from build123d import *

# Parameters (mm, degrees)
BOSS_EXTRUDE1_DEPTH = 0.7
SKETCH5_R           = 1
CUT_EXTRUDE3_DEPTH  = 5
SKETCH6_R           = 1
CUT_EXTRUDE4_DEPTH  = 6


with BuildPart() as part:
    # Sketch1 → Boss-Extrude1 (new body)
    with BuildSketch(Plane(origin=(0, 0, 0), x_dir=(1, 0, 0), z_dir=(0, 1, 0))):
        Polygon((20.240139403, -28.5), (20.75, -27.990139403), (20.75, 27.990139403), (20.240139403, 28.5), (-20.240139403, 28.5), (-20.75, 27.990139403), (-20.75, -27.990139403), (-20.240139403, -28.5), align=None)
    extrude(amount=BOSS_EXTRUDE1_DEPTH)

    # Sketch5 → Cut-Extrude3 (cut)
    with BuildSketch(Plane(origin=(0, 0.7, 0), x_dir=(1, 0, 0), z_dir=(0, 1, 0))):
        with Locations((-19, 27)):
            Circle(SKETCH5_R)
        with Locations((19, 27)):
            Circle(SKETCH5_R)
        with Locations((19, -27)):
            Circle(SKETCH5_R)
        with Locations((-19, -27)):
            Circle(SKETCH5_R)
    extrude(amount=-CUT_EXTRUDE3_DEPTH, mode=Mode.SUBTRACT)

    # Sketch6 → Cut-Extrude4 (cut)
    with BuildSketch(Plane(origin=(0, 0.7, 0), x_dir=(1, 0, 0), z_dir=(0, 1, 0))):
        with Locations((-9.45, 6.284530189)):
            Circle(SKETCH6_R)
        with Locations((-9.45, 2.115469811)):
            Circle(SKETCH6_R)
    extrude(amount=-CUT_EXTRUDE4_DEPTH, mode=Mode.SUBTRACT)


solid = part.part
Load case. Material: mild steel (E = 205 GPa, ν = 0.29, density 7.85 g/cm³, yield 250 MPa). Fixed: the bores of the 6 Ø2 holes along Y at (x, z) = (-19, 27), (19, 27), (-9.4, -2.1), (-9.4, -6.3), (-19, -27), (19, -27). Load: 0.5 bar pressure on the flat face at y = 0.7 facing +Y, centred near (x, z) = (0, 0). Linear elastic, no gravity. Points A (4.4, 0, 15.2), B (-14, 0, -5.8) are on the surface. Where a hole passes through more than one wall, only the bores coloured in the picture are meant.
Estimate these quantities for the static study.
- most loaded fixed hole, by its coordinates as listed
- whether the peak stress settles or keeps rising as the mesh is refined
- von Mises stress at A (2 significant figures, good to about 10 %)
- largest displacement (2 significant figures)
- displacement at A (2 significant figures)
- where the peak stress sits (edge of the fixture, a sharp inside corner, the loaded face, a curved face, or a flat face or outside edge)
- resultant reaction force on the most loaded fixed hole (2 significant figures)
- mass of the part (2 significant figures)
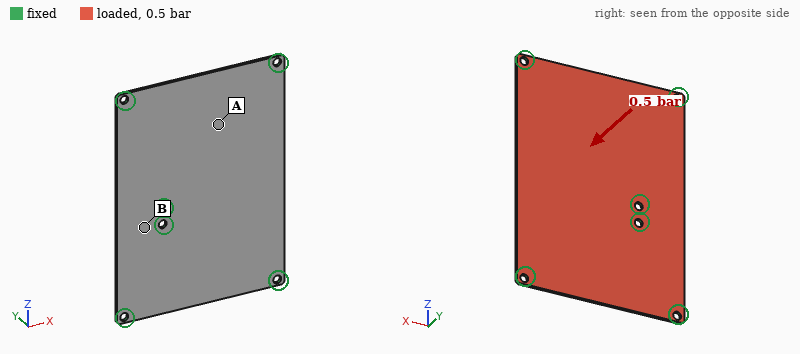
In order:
(-9.4, -2.1)
keeps rising
46 MPa
0.16 mm
0.079 mm
edge of the fixture
34 N
13 g
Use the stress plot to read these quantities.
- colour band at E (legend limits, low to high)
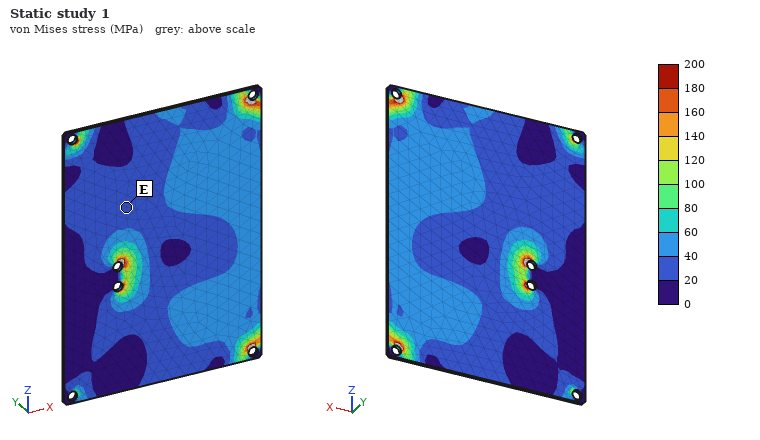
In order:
20 to 40 MPa
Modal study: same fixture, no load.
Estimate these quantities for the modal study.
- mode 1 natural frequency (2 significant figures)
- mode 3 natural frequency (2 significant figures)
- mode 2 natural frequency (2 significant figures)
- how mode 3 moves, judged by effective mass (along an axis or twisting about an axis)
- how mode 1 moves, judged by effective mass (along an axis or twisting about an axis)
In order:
1600 Hz
2900 Hz
2500 Hz
along Y
along Y
